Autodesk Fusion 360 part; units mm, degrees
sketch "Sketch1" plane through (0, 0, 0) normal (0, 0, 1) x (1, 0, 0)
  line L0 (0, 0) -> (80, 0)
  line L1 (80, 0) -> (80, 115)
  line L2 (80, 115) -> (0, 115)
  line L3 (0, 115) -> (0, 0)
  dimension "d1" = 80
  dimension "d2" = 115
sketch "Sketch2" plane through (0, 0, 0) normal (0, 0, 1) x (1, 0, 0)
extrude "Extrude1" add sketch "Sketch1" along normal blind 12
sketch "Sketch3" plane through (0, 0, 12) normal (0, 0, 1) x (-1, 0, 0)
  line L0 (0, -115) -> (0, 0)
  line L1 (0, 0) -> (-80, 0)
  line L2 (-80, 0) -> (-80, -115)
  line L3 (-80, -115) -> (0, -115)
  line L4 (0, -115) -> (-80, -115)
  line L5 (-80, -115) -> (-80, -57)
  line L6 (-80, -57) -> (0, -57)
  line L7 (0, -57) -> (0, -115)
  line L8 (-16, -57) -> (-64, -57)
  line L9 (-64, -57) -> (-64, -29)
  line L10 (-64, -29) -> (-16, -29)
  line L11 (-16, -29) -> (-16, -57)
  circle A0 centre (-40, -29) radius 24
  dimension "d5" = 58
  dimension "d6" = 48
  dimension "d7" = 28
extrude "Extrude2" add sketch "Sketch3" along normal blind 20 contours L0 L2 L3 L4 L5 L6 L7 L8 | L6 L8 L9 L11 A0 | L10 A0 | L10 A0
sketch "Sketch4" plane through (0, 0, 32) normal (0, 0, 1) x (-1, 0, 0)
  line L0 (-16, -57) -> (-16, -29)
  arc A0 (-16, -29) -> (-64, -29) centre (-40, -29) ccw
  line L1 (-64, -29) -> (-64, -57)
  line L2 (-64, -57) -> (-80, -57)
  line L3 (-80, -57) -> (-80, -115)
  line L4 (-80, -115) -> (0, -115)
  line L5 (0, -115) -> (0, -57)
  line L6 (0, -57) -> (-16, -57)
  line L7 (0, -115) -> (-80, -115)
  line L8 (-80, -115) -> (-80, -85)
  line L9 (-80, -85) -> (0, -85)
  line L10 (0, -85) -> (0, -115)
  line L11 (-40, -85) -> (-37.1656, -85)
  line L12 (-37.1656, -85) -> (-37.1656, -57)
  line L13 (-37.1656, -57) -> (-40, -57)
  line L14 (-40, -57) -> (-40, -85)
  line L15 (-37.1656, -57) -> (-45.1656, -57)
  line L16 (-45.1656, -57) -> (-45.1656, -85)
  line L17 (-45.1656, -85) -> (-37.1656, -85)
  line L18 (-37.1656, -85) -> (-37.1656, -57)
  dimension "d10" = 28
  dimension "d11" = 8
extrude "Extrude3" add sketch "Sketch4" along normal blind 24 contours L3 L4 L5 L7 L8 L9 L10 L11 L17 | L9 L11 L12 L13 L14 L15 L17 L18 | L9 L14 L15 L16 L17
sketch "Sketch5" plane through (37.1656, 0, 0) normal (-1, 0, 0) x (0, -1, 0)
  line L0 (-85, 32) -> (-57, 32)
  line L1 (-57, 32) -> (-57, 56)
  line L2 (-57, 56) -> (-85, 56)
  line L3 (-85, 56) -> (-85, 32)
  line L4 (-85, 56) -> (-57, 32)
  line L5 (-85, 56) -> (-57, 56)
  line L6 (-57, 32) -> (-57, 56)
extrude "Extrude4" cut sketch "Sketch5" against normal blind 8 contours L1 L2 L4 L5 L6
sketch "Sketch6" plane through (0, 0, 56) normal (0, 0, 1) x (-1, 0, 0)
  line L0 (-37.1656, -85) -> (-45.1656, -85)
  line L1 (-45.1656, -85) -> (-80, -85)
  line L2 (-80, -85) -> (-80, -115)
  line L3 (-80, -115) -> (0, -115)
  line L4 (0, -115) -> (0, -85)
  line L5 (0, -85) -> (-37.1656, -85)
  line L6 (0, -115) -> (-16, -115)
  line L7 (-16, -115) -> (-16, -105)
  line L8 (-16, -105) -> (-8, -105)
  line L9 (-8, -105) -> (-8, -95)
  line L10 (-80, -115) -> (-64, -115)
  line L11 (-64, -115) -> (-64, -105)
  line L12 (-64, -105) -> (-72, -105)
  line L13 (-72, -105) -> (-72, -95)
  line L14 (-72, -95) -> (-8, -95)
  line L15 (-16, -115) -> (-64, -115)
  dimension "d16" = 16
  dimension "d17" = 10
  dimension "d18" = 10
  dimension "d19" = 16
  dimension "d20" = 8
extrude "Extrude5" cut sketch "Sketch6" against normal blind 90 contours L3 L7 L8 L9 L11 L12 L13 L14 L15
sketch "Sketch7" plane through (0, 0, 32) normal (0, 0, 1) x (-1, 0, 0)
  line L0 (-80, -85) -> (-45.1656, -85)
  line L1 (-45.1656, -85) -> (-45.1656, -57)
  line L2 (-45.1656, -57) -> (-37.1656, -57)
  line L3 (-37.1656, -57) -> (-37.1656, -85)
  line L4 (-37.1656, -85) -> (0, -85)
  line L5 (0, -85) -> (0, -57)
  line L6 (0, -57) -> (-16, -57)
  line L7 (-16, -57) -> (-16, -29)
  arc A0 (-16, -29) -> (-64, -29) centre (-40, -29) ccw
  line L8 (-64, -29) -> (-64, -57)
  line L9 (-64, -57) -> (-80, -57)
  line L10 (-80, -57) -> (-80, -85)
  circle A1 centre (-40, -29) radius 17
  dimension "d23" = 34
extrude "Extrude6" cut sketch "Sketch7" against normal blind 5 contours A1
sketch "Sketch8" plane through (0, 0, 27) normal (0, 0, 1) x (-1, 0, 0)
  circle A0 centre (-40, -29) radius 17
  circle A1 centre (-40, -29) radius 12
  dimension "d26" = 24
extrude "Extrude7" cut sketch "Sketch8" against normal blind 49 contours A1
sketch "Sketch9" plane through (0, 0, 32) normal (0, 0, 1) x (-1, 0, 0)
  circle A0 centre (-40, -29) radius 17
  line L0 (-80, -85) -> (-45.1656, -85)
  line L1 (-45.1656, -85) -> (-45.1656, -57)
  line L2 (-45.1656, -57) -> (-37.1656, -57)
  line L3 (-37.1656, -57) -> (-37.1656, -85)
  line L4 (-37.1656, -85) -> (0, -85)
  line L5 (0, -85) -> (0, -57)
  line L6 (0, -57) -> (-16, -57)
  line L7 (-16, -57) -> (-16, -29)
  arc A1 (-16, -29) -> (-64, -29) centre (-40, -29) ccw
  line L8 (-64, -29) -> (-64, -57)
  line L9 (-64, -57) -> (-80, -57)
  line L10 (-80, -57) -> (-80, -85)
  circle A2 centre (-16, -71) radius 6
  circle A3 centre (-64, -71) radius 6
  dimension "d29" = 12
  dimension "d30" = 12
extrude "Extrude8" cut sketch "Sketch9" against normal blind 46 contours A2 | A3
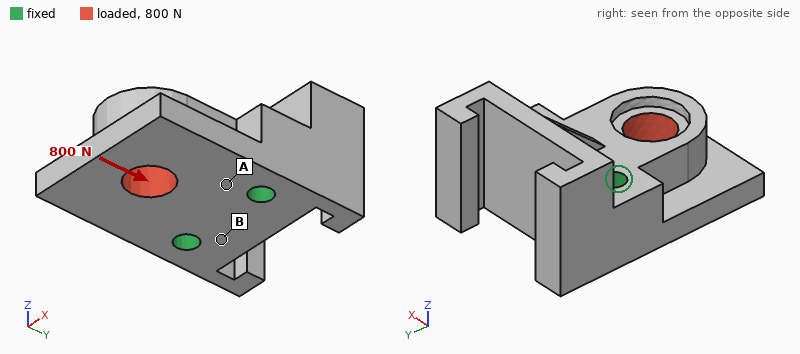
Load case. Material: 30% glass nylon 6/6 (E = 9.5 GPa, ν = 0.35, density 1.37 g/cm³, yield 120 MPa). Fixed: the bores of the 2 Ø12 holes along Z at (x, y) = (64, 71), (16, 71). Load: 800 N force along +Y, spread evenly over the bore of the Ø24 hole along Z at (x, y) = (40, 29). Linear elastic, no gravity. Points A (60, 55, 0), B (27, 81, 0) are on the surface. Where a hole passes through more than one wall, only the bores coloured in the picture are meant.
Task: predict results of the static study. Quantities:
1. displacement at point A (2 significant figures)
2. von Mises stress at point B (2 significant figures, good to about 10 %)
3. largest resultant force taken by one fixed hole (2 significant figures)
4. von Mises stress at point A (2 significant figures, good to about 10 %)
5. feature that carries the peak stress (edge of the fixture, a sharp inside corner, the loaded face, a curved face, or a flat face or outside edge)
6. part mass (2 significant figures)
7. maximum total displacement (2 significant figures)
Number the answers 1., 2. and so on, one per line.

1. 0.93 µm
2. 0.22 MPa
3. 410 N
4. 0.63 MPa
5. the loaded face
6. 300 g
7. 4.4 µm
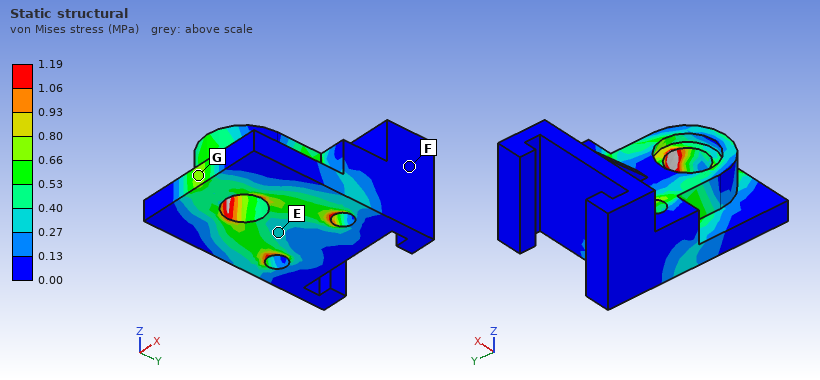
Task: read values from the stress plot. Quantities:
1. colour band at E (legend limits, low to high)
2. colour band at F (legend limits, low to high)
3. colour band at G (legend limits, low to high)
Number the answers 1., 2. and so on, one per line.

1. 0.27 to 0.40 MPa
2. 0.00 to 0.13 MPa
3. 0.66 to 0.80 MPa
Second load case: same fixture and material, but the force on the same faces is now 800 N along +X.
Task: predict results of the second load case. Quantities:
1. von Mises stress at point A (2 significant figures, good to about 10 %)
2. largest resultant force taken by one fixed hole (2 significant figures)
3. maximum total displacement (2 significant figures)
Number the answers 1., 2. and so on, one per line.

1. 0.75 MPa
2. 720 N
3. 16 µm
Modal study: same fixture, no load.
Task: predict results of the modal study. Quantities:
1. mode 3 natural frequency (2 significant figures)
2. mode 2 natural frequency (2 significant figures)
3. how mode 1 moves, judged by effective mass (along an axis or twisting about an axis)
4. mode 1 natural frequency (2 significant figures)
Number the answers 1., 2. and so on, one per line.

1. 3400 Hz
2. 3300 Hz
3. along Z
4. 2600 Hz
